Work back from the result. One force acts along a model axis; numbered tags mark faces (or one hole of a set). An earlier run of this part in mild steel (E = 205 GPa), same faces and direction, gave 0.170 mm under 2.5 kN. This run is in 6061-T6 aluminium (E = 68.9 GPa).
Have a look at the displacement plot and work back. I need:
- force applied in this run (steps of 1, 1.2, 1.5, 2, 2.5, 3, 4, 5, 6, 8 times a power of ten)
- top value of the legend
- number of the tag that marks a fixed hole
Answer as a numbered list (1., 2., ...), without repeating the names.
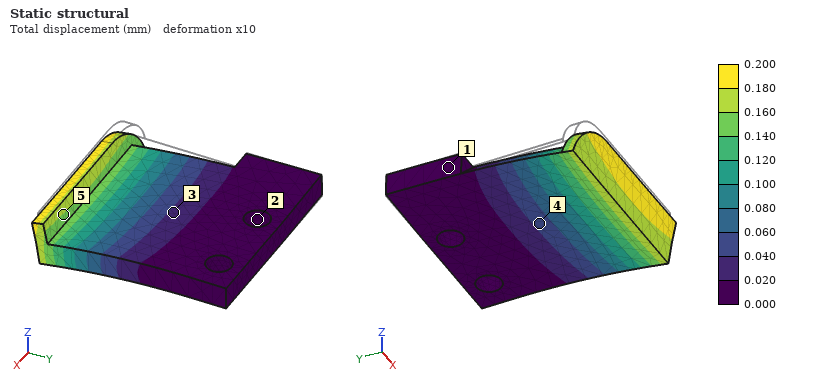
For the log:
1. 1 kN
2. 0.200 mm
3. 2
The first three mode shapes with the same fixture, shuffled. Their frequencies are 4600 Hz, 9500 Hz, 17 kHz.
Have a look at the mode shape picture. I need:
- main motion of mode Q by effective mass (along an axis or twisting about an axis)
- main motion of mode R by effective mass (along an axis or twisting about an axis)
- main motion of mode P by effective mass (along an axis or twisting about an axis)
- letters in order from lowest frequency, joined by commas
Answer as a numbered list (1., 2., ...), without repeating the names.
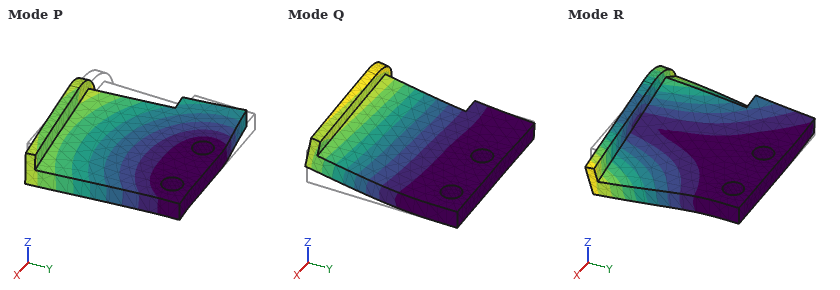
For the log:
1. along Z
2. twisting about Y
3. along X
4. Q, R, P
